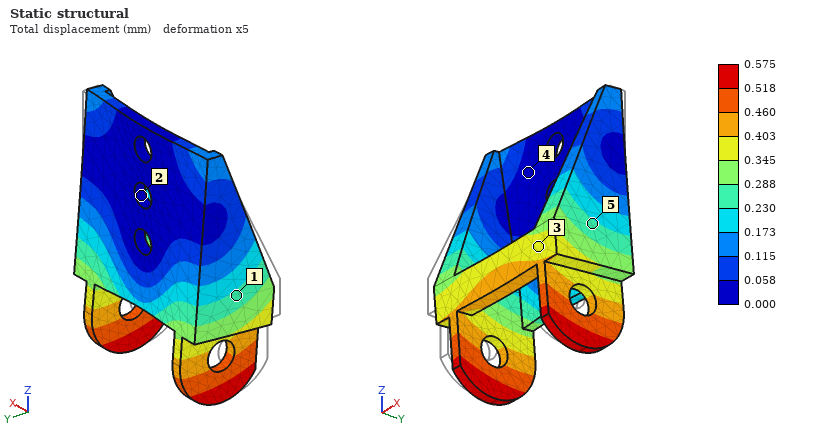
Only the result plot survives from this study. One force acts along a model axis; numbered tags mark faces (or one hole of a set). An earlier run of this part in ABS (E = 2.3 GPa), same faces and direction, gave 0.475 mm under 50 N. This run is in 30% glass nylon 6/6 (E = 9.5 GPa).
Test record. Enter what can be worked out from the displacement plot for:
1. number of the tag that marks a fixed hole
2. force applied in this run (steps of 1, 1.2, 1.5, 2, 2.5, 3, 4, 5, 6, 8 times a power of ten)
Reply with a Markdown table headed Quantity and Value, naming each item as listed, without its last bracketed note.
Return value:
| Quantity | Value |
|---|---|
| number of the tag that marks a fixed hole | 2 |
| force applied in this run | 250 N |
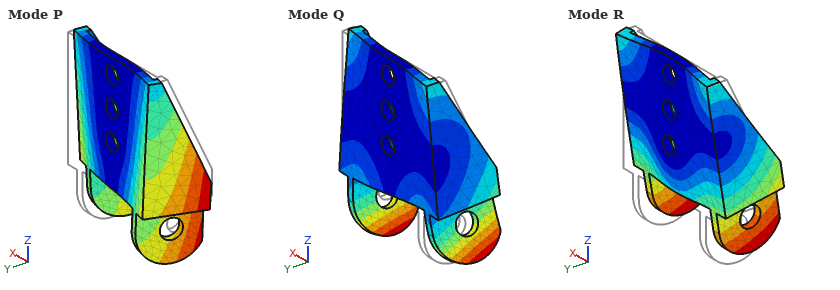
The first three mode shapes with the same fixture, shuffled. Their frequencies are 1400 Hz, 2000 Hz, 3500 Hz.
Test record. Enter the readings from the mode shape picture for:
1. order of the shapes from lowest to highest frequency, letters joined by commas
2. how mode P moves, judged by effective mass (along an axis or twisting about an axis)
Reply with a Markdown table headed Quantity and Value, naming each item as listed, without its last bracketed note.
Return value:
| Quantity | Value |
|---|---|
| order of the shapes from lowest to highest frequency, letters joined by commas | P, R, Q |
| how mode P moves, judged by effective mass | along X |
